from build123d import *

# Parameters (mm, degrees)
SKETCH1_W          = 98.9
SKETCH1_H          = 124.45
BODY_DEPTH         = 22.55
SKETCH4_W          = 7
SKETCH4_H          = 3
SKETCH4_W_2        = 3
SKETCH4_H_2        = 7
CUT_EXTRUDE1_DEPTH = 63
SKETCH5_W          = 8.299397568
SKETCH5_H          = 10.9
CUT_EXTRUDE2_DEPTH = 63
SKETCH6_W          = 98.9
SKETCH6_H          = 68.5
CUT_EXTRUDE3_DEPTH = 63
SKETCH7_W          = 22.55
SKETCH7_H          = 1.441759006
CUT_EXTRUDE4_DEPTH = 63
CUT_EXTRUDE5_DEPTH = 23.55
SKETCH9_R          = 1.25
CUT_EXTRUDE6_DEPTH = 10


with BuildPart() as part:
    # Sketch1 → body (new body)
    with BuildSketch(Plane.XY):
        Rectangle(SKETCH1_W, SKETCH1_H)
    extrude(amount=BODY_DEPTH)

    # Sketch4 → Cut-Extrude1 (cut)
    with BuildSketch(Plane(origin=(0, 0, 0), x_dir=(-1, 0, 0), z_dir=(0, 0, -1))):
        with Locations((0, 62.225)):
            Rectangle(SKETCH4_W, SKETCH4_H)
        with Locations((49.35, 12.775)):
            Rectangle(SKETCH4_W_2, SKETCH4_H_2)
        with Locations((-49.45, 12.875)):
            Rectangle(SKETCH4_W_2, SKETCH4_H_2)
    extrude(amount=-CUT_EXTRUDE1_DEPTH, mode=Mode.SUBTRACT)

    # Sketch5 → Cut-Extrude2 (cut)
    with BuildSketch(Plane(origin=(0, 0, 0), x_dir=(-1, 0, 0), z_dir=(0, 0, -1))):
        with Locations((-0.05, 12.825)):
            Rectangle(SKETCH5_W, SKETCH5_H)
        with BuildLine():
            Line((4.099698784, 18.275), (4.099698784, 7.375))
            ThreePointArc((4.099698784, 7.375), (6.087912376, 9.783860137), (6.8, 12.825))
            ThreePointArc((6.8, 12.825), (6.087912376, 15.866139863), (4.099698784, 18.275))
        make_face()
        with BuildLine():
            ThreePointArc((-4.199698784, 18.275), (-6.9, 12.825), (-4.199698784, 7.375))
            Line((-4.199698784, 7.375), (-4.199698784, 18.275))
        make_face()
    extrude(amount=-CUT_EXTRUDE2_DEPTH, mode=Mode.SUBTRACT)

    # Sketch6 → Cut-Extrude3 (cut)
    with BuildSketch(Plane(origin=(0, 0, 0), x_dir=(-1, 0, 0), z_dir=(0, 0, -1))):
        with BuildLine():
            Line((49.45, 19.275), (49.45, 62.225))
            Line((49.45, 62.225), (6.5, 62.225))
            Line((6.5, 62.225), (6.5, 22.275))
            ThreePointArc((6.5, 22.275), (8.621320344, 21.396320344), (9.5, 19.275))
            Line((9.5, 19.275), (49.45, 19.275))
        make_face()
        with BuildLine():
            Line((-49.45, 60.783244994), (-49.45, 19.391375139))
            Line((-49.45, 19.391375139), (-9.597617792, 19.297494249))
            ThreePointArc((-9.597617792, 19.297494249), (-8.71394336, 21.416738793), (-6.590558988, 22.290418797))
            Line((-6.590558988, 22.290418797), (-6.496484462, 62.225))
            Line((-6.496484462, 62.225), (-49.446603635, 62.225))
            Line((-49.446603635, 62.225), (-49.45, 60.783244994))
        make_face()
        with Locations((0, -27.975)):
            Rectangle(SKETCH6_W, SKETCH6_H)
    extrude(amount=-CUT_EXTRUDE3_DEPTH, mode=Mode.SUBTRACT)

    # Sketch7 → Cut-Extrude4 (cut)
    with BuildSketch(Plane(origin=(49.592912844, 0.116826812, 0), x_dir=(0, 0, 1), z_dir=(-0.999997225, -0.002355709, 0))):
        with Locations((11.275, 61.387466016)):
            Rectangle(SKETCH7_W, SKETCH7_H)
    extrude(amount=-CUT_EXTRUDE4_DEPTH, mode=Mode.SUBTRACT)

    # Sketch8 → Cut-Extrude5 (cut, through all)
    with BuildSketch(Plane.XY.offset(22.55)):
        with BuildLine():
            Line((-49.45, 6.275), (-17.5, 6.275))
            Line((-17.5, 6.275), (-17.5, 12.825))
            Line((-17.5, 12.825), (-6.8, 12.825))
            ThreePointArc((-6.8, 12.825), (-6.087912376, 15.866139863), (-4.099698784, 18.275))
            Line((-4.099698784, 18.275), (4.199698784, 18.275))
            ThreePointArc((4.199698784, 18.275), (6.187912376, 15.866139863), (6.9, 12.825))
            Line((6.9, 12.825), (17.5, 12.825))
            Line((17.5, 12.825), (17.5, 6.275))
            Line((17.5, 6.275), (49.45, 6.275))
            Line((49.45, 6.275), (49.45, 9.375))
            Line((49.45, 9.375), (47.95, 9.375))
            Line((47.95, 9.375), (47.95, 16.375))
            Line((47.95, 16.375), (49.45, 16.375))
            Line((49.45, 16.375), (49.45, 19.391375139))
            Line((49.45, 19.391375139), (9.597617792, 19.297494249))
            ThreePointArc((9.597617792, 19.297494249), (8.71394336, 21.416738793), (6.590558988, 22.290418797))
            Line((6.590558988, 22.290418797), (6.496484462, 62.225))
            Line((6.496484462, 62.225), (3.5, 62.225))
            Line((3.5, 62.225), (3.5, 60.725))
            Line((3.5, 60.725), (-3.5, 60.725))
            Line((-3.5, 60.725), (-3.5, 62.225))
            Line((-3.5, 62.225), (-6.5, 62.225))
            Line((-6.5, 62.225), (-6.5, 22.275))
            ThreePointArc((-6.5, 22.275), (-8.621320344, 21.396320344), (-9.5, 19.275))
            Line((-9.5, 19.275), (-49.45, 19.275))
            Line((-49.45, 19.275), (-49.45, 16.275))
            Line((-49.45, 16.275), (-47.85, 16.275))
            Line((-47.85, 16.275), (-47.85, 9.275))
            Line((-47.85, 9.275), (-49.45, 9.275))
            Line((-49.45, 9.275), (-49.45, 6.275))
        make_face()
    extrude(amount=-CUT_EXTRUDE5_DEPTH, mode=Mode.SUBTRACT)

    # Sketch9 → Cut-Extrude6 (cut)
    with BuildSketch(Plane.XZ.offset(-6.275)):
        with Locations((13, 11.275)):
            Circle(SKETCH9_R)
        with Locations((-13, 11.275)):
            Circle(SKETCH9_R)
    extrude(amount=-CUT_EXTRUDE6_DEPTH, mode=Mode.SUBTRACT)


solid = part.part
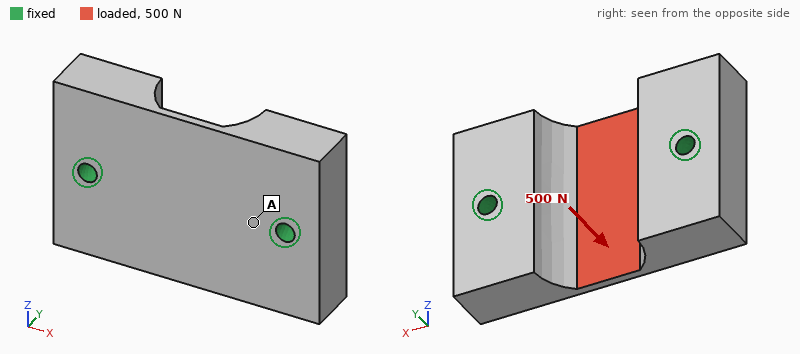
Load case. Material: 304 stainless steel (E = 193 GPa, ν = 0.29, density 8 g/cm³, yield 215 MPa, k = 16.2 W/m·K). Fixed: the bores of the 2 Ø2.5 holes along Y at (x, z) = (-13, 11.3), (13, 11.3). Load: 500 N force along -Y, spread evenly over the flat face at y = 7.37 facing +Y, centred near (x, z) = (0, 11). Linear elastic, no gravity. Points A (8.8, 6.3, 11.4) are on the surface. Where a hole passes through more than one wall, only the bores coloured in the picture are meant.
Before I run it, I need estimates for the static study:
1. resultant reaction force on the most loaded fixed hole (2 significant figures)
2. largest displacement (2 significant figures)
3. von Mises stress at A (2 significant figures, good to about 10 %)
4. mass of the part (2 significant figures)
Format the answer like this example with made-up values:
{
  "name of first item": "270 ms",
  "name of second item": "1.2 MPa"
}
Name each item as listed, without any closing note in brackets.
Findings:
{
  "resultant reaction force on the most loaded fixed hole": "370 N",
  "largest displacement": "5.9 µm",
  "von Mises stress at A": "9.5 MPa",
  "mass of the part": "29 g"
}
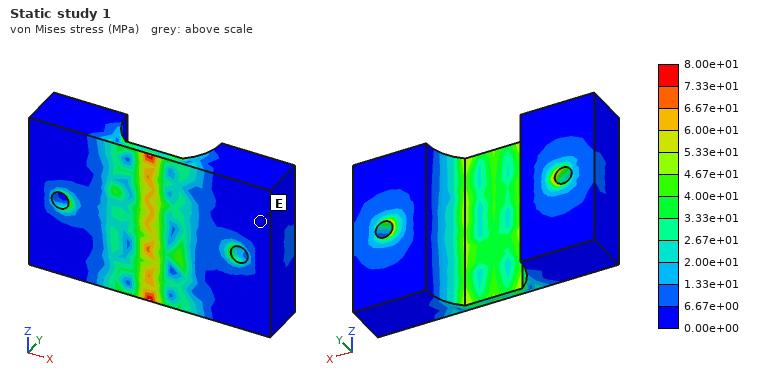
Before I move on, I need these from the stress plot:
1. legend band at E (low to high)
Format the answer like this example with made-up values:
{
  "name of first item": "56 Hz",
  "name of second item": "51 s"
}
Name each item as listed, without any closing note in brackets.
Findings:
{
  "legend band at E": "0.00e+00 to 6.67e+00 MPa"
}
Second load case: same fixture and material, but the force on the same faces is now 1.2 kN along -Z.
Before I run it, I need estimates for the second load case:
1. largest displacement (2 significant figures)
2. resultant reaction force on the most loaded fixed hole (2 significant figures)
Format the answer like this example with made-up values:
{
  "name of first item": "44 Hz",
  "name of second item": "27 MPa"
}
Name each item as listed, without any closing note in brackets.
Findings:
{
  "largest displacement": "4.1 µm",
  "resultant reaction force on the most loaded fixed hole": "600 N"
}
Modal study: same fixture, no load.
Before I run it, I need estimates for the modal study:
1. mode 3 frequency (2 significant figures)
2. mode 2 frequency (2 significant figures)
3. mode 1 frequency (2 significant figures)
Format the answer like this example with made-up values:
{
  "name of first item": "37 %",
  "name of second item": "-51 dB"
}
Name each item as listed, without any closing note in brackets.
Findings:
{
  "mode 3 frequency": "30 kHz",
  "mode 2 frequency": "26 kHz",
  "mode 1 frequency": "24 kHz"
}
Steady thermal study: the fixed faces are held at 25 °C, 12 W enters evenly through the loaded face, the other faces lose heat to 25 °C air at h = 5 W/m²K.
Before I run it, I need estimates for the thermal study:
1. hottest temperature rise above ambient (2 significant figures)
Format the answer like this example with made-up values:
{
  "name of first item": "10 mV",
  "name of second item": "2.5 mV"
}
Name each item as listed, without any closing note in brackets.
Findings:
{
  "hottest temperature rise above ambient": "86 K"
}
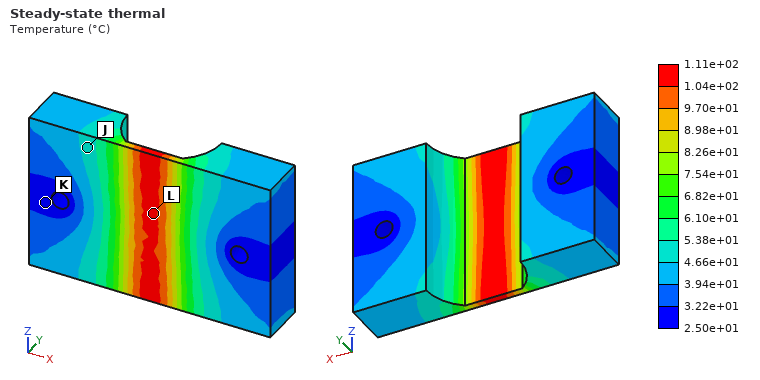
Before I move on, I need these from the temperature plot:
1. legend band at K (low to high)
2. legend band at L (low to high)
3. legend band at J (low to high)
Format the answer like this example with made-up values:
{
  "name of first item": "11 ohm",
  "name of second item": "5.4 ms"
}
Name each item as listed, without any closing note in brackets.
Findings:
{
  "legend band at K": "2.50e+01 to 3.22e+01 °C",
  "legend band at L": "1.04e+02 to 1.11e+02 °C",
  "legend band at J": "4.66e+01 to 5.38e+01 °C"
}
